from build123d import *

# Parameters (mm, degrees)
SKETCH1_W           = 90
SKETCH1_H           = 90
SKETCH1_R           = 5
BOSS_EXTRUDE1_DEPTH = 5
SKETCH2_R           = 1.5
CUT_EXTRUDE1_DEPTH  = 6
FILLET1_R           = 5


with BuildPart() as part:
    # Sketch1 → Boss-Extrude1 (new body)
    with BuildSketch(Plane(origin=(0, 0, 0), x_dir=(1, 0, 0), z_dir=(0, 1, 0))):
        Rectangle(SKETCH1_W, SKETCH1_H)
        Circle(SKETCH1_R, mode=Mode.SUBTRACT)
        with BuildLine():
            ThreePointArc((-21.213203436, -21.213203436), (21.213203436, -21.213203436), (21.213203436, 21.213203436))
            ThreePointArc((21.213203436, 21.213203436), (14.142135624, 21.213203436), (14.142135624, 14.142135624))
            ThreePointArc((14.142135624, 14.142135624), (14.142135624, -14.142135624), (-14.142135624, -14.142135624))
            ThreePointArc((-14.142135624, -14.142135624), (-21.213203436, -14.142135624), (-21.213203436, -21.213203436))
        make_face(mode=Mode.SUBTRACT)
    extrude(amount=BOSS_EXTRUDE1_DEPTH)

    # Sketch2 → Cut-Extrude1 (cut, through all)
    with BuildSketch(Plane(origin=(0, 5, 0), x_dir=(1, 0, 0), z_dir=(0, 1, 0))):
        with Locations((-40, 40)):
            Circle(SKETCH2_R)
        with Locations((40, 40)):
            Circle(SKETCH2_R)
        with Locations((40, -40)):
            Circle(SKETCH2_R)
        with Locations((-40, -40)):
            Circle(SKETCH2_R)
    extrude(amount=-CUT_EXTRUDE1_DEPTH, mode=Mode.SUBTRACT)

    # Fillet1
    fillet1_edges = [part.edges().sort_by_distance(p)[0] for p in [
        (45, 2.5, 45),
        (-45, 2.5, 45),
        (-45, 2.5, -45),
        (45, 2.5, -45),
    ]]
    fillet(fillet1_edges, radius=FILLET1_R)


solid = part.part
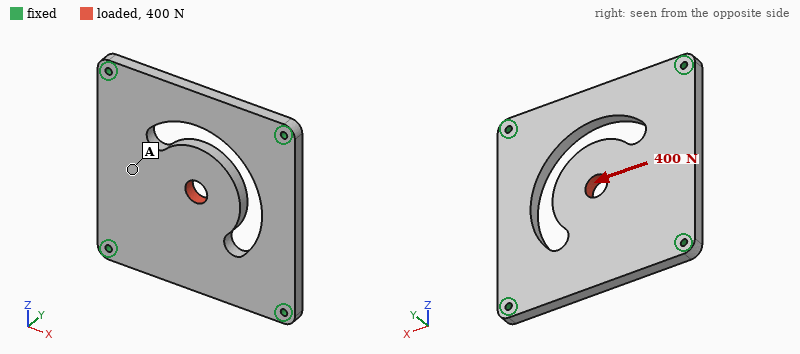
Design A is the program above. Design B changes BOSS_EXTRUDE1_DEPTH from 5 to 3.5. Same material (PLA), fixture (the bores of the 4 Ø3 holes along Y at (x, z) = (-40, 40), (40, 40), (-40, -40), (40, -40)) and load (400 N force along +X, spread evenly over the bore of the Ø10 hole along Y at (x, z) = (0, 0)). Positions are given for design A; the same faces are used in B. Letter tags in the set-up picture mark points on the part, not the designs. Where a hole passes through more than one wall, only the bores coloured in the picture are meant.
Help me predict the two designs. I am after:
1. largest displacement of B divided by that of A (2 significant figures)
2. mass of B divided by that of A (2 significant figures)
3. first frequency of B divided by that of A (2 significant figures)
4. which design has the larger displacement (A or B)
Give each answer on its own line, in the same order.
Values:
1.4
0.70
0.73
B
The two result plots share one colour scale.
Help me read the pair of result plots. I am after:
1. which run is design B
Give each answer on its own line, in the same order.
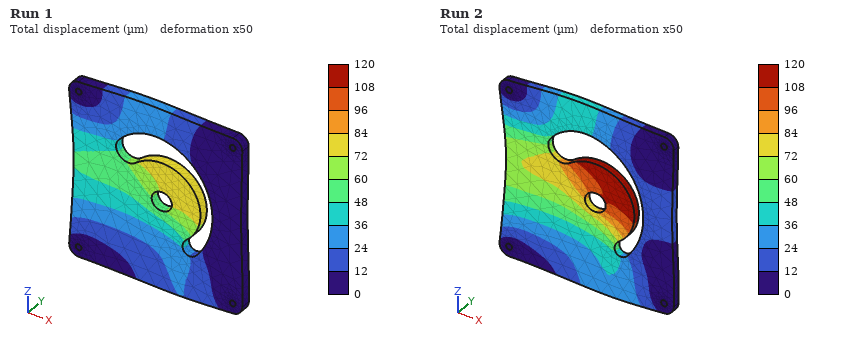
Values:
Run 2
